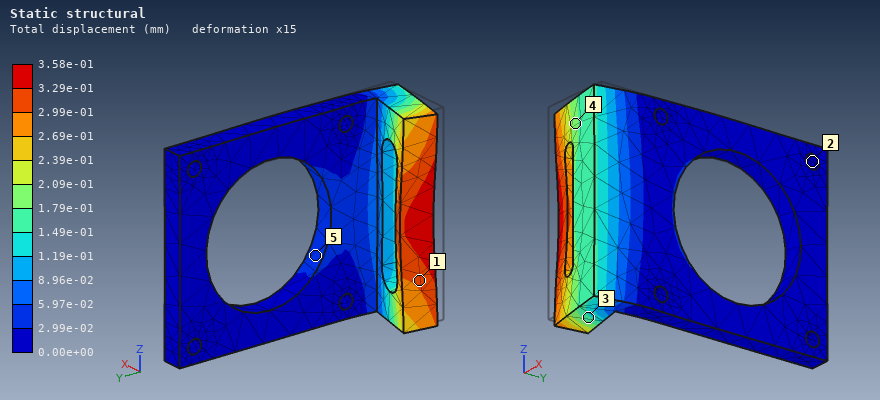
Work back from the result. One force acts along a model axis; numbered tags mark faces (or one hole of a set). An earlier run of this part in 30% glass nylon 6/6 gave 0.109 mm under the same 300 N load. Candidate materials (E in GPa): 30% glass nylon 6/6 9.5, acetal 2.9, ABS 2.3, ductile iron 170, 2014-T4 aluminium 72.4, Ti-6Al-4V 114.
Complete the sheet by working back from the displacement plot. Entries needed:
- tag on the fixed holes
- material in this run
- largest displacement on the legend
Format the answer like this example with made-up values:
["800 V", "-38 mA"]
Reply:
["2", "acetal", "3.58e-01 mm"]
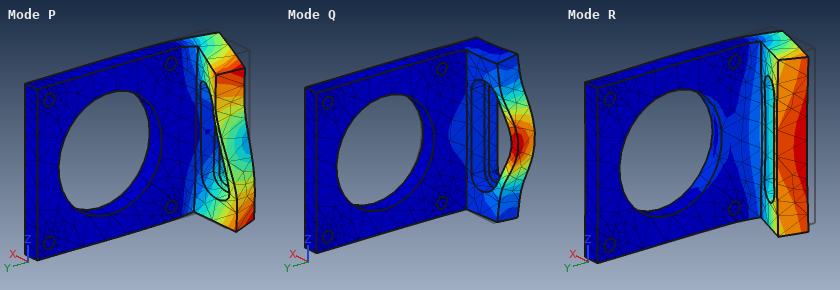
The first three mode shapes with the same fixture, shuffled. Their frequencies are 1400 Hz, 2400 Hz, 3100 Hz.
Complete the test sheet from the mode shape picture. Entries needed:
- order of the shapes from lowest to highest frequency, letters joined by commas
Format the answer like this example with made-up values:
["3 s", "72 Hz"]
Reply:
["R, P, Q"]
